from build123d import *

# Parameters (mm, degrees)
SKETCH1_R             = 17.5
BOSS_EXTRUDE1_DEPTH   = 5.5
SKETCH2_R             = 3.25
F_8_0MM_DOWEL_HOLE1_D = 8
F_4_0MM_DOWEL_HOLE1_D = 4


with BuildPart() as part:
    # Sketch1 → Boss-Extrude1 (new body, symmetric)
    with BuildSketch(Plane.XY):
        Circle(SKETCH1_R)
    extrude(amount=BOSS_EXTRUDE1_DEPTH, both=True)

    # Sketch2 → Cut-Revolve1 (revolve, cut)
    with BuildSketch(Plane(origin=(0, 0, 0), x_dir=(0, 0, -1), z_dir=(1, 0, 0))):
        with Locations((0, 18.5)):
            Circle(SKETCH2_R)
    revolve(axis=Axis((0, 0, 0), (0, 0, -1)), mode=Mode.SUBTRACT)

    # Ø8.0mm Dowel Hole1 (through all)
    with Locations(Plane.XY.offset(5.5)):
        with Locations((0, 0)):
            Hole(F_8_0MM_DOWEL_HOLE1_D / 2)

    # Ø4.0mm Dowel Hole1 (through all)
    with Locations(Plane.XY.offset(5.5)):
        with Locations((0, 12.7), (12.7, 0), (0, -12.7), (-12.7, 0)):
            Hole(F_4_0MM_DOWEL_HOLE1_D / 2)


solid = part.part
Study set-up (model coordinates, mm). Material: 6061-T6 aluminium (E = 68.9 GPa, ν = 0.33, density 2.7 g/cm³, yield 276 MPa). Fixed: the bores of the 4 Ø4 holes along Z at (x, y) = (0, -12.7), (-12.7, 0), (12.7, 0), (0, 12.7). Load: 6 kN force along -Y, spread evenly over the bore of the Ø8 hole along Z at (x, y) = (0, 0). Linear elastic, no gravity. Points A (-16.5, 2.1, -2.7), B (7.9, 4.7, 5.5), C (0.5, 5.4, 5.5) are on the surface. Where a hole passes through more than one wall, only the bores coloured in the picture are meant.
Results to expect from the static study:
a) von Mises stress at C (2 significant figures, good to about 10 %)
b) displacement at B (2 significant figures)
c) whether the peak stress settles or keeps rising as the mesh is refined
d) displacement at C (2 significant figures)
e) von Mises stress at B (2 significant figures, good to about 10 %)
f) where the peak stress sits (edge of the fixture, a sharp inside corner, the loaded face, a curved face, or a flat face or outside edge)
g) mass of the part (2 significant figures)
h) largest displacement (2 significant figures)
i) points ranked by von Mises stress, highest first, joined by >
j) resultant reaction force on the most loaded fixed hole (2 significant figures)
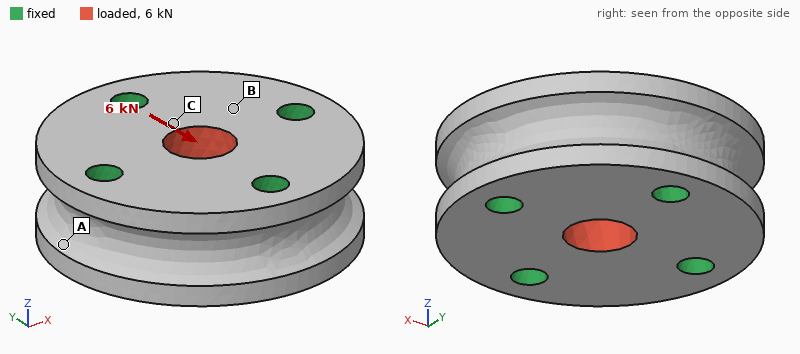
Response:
26 MPa
1.3 µm
keeps rising
2.2 µm
7.3 MPa
edge of the fixture
23 g
3.1 µm
C > B > A
2.0 kN
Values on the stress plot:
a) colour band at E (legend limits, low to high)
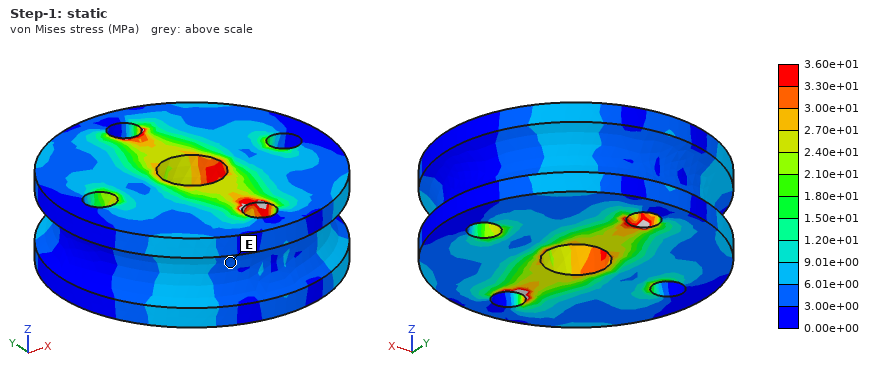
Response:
3.00e+00 to 6.01e+00 MPa
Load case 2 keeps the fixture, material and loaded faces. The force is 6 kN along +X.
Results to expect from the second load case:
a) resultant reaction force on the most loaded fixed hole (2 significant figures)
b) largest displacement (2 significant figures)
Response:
2.0 kN
3.1 µm
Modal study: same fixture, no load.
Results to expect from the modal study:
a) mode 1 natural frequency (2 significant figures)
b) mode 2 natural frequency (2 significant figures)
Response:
63 kHz
65 kHz
